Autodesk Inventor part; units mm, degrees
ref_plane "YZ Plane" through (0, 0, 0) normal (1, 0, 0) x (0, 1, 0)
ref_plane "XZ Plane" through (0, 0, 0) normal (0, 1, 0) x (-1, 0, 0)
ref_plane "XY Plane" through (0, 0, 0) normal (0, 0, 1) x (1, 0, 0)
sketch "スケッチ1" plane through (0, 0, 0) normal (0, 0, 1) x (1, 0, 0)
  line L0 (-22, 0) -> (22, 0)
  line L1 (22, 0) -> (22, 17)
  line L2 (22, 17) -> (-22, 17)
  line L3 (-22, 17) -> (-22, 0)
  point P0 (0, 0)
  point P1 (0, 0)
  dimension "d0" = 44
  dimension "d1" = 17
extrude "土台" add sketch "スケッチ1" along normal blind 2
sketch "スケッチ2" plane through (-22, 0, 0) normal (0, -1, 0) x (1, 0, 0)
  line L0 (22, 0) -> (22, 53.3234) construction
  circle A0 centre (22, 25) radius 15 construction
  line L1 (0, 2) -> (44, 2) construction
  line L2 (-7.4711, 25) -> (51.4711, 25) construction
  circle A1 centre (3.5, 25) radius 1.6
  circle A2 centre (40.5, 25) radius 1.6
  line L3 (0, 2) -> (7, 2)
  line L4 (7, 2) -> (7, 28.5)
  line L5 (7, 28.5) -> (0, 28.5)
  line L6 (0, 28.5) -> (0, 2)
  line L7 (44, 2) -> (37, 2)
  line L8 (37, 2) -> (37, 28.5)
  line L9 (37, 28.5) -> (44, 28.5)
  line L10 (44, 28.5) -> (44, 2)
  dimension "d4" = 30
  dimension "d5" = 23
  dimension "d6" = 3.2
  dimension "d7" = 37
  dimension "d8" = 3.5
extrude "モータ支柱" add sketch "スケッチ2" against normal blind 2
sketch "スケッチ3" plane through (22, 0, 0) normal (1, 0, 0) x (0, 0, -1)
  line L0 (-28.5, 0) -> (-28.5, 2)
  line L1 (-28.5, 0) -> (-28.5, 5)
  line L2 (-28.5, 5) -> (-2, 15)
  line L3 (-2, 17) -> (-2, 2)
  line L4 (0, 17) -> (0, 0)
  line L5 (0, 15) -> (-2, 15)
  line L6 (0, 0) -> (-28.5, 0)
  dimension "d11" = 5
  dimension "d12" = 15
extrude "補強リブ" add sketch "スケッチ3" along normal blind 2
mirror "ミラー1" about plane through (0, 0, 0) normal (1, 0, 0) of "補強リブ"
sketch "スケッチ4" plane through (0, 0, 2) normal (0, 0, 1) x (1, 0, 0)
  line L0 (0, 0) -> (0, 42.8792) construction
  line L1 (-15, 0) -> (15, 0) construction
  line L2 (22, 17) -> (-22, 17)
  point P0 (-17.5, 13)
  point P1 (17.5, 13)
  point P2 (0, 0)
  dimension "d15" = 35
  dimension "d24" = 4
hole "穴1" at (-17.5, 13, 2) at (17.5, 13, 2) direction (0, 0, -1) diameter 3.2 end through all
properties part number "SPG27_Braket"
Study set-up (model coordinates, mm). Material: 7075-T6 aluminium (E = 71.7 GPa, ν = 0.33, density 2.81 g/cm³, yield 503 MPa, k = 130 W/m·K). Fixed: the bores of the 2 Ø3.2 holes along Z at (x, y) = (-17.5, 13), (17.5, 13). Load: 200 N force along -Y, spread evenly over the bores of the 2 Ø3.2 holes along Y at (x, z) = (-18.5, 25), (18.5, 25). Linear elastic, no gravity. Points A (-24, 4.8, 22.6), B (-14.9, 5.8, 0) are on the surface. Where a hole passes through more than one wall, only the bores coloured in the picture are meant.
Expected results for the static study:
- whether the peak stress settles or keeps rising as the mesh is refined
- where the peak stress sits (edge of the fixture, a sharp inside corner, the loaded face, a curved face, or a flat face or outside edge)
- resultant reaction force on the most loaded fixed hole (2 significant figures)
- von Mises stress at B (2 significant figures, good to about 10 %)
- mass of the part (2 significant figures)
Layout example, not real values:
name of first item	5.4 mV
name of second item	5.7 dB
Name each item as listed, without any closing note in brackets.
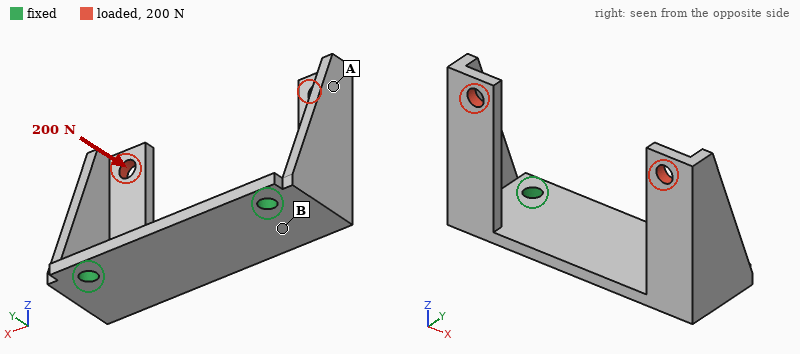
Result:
whether the peak stress settles or keeps rising as the mesh is refined	keeps rising
where the peak stress sits	edge of the fixture
resultant reaction force on the most loaded fixed hole	100 N
von Mises stress at B	69 MPa
mass of the part	9.4 g
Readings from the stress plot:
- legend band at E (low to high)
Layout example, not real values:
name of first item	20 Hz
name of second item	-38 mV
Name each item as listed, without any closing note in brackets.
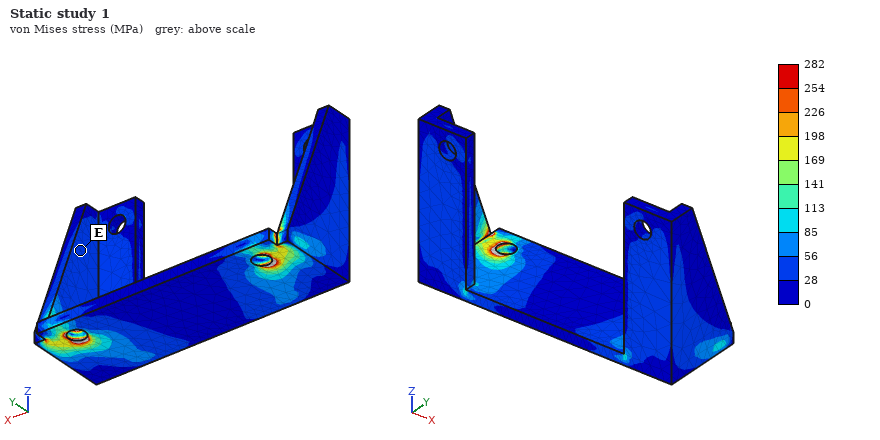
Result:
legend band at E	28 to 56 MPa
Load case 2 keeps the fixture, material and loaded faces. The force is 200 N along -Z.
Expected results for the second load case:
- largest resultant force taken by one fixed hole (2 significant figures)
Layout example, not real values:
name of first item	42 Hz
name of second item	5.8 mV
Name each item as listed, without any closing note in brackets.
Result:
largest resultant force taken by one fixed hole	100 N
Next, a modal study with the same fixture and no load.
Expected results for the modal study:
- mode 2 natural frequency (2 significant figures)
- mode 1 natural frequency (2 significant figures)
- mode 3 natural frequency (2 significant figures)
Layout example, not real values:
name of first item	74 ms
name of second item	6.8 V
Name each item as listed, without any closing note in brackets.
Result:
mode 2 natural frequency	2200 Hz
mode 1 natural frequency	2200 Hz
mode 3 natural frequency	3100 Hz
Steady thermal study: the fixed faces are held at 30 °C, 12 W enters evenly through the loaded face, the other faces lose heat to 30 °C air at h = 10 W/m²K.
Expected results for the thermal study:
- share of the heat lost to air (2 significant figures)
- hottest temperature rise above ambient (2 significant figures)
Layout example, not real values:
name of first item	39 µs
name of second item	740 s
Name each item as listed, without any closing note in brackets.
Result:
share of the heat lost to air	5.4 %
hottest temperature rise above ambient	51 K
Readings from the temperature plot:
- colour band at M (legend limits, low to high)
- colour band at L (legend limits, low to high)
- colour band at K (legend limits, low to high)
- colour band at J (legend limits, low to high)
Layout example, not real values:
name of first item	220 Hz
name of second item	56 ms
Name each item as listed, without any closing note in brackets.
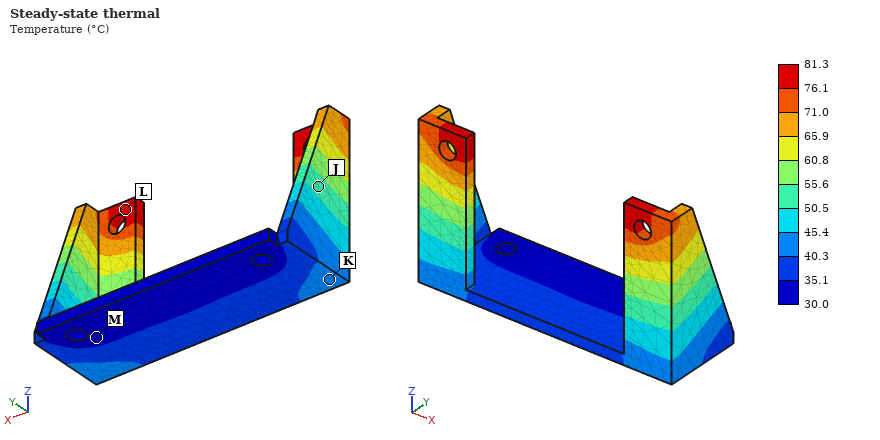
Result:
colour band at M	30.0 to 35.1 °C
colour band at L	76.1 to 81.3 °C
colour band at K	40.3 to 45.4 °C
colour band at J	50.5 to 55.6 °C
